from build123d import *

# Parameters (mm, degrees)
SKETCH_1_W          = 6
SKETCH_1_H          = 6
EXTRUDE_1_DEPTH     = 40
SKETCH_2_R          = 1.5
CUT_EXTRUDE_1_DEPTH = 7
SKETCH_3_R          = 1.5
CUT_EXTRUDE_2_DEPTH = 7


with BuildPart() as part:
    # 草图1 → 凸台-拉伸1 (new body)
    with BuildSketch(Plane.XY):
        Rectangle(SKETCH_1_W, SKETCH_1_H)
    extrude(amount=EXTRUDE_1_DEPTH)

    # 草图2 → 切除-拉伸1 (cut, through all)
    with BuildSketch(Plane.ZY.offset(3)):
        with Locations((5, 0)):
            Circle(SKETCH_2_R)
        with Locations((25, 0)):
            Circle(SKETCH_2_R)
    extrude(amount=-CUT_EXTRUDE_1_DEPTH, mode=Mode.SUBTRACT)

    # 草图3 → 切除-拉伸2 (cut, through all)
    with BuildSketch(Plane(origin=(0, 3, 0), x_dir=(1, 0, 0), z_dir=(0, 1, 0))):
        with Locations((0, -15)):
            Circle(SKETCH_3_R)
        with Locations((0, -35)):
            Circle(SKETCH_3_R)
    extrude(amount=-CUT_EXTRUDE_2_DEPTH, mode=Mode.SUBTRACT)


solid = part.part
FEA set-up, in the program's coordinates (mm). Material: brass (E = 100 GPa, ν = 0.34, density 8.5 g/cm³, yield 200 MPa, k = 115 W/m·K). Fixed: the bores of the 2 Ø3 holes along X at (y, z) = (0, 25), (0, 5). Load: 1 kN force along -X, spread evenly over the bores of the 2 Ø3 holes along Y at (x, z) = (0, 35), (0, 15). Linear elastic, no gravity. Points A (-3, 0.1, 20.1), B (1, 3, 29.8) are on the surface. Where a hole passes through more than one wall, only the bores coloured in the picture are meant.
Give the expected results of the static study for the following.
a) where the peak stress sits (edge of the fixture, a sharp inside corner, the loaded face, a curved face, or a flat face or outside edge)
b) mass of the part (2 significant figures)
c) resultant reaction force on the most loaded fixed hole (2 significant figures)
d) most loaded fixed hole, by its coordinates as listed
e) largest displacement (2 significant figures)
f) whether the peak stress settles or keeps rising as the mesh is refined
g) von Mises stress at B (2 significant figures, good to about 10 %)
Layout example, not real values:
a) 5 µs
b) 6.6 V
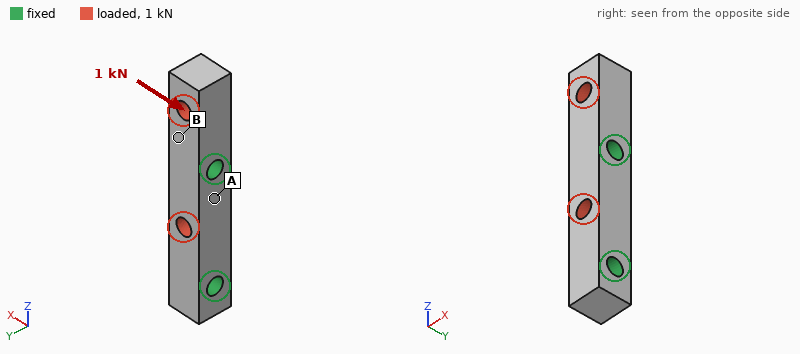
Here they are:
a) edge of the fixture
b) 11 g
c) 760 N
d) (0, 25)
e) 29 µm
f) keeps rising
g) 40 MPa
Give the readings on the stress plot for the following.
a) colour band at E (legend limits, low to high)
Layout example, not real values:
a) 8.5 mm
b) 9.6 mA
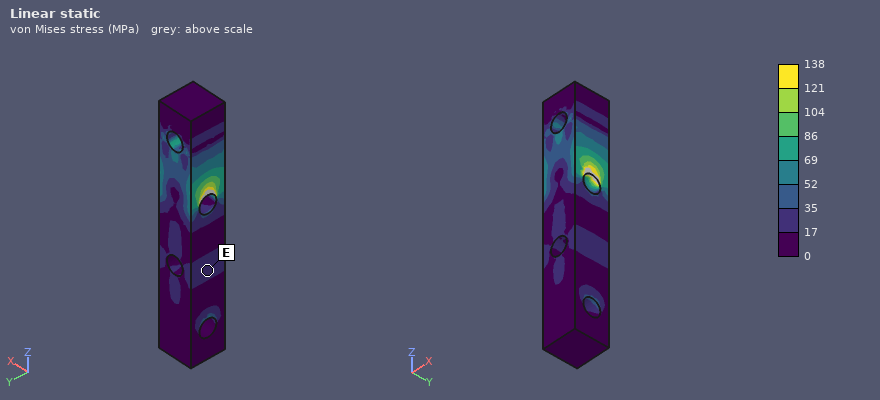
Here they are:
a) 17 to 35 MPa
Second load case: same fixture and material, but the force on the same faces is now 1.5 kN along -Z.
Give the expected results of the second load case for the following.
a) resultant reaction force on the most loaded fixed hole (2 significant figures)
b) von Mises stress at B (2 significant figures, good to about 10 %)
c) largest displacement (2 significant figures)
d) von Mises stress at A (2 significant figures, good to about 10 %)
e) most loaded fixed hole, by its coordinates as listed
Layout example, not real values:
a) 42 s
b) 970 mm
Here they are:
a) 1.1 kN
b) 18 MPa
c) 2.8 µm
d) 11 MPa
e) (0, 25)
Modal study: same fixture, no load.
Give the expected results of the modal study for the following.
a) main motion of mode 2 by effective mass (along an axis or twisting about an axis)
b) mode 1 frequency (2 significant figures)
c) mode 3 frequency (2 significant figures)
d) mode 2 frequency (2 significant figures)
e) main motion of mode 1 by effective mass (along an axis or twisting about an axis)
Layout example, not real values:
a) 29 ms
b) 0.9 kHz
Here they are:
a) along X
b) 13 kHz
c) 33 kHz
d) 15 kHz
e) along Y
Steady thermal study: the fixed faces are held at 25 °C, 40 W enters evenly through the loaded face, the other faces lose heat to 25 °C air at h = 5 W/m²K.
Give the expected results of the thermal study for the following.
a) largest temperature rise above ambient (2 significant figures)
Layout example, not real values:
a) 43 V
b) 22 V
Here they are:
a) 53 K
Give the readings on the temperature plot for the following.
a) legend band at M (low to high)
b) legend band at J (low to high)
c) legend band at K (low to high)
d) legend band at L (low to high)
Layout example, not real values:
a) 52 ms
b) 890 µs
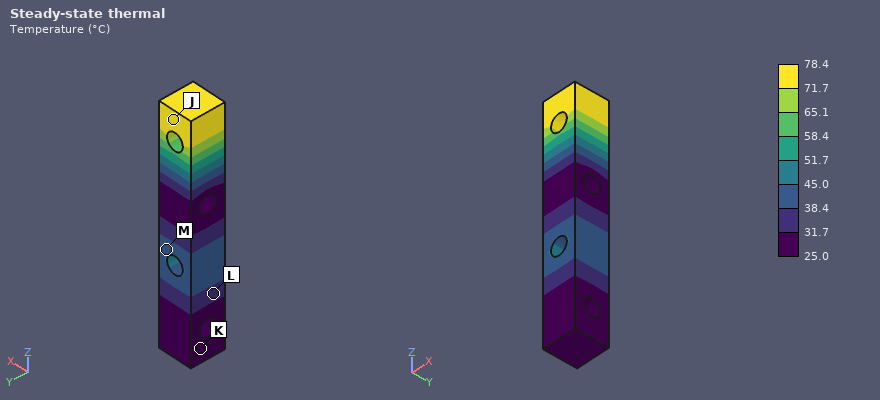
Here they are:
a) 38.4 to 45.0 °C
b) 71.7 to 78.4 °C
c) 25.0 to 31.7 °C
d) 31.7 to 38.4 °C
